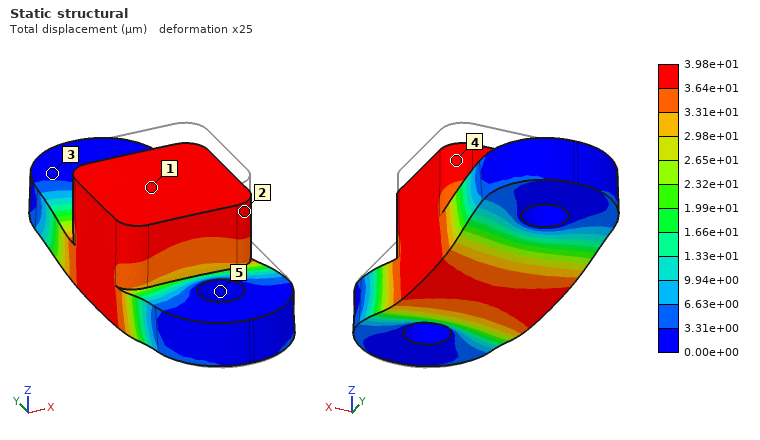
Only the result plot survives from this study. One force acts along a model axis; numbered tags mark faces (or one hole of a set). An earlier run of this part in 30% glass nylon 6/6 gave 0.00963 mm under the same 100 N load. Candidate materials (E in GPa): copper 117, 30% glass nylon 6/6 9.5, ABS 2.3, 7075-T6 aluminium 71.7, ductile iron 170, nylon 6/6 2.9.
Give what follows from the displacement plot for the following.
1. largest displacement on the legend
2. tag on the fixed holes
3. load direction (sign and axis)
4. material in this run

3.98e+01 µm
5
-Z
ABS
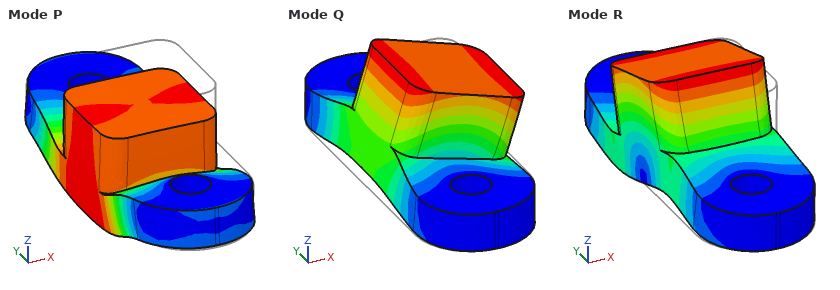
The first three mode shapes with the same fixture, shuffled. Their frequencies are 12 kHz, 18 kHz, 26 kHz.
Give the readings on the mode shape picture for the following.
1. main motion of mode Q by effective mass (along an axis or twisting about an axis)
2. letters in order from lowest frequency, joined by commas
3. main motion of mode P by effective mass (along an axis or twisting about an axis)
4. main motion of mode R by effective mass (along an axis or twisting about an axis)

along X
Q, P, R
along Z
along Y
